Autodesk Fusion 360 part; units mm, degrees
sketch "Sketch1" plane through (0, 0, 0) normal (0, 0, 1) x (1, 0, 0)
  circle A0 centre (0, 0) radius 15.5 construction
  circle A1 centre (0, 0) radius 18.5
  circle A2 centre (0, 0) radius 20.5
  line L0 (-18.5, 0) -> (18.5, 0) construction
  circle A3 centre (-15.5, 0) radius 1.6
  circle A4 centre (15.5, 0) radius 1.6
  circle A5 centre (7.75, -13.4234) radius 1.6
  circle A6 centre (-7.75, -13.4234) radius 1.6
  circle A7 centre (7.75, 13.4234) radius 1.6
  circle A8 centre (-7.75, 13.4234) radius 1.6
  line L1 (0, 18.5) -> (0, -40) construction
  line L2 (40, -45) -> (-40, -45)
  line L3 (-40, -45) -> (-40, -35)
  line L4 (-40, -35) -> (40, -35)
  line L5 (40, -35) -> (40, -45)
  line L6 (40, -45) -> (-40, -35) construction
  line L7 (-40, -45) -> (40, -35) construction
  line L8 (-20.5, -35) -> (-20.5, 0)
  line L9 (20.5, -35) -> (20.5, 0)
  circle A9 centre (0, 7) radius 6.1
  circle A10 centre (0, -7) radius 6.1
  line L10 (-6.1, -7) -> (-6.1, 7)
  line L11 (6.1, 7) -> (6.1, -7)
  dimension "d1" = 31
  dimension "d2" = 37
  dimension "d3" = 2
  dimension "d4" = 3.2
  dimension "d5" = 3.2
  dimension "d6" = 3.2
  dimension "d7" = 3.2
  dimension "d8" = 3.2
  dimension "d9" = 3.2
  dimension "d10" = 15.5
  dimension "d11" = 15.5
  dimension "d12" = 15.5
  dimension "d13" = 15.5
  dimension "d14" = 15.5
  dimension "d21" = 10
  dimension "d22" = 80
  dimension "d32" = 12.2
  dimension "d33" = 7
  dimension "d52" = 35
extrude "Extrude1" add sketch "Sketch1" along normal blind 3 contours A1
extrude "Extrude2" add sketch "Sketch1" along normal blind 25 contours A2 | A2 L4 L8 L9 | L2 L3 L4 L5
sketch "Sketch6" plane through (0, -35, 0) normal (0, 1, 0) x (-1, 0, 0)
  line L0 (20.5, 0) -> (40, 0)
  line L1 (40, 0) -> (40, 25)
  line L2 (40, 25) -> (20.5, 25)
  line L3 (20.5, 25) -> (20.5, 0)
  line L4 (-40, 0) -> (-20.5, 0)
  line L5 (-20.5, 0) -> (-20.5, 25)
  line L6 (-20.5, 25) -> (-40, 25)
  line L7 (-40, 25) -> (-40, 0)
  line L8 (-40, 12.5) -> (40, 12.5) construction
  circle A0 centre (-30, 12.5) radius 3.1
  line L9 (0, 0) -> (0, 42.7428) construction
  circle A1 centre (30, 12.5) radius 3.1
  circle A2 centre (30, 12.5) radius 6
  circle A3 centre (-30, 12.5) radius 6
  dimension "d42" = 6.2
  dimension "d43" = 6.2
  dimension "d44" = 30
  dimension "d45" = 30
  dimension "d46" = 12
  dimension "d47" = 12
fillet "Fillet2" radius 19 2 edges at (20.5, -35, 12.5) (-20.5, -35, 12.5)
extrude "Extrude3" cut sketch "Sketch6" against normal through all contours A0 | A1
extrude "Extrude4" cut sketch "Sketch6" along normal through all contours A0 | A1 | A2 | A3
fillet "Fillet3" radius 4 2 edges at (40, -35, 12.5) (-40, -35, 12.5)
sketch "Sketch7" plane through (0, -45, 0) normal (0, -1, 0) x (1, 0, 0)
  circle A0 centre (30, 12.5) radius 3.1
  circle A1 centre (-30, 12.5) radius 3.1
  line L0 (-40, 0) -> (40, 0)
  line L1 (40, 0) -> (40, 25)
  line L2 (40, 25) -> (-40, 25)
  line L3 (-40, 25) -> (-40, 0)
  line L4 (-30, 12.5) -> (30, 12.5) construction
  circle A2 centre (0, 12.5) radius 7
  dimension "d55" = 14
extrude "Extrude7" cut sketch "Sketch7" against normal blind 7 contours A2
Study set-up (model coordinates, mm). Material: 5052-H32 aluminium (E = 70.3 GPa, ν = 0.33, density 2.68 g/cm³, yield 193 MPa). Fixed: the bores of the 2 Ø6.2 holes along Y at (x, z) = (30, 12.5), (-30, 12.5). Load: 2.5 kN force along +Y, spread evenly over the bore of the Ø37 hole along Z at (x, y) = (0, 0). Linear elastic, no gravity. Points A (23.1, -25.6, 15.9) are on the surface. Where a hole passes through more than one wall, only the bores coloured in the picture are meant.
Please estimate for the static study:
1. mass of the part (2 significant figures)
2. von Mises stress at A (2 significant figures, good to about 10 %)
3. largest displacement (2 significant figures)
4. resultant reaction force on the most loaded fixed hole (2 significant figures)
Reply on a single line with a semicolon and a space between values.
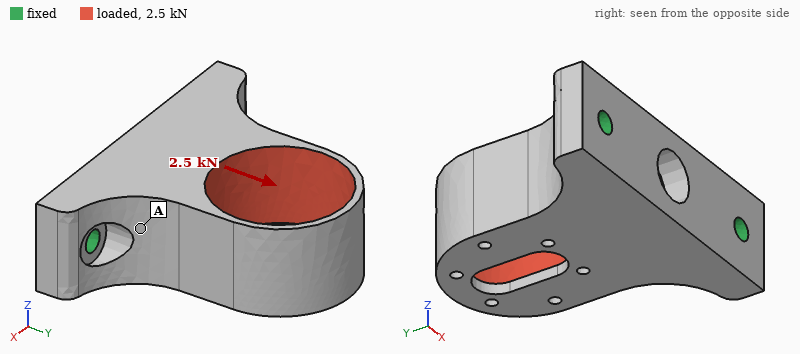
130 g; 9.8 MPa; 85 µm; 1.4 kN
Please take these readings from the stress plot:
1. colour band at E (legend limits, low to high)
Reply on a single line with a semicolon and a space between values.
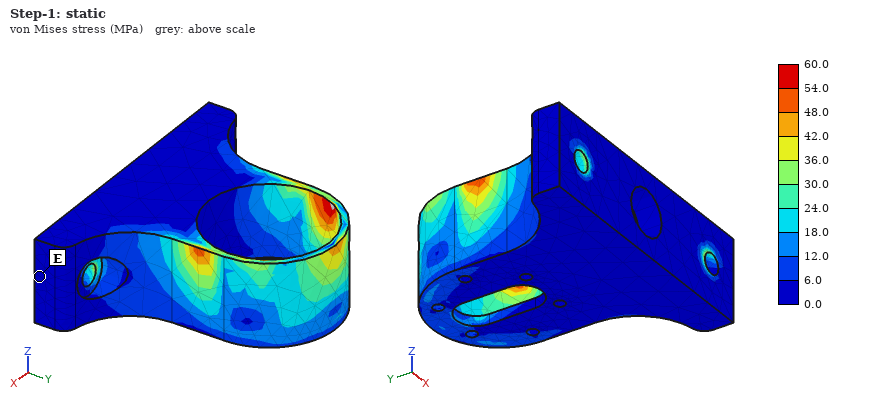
0.0 to 6.0 MPa
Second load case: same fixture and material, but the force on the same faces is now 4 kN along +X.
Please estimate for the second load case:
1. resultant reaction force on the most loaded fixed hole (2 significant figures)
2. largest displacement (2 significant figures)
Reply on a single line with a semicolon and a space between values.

3.5 kN; 0.24 mm
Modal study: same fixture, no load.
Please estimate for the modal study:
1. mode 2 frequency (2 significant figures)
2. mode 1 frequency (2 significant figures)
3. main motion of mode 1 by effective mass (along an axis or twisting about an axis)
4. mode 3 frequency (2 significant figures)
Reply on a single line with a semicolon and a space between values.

5900 Hz; 3900 Hz; along Z; 7800 Hz
